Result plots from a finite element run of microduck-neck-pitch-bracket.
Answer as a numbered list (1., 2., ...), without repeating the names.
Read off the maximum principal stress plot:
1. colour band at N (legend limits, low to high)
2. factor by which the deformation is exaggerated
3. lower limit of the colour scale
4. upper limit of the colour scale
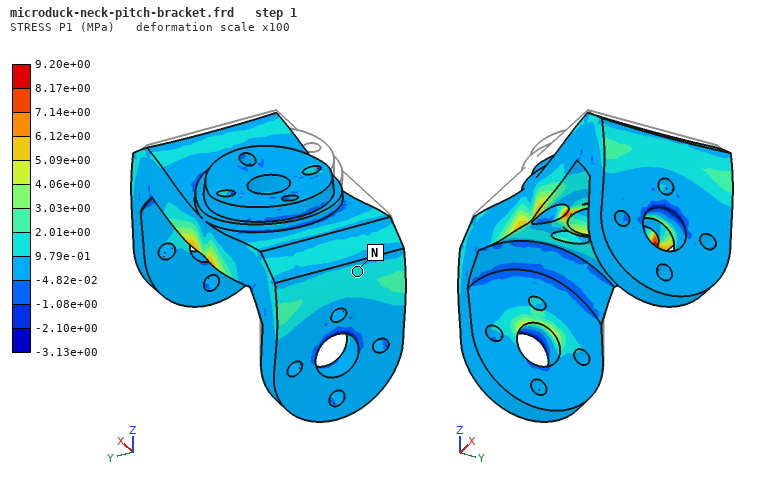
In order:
1. 9.79e-01 to 2.01e+00 MPa
2. 100
3. -3.13e+00 MPa
4. 9.20e+00 MPa
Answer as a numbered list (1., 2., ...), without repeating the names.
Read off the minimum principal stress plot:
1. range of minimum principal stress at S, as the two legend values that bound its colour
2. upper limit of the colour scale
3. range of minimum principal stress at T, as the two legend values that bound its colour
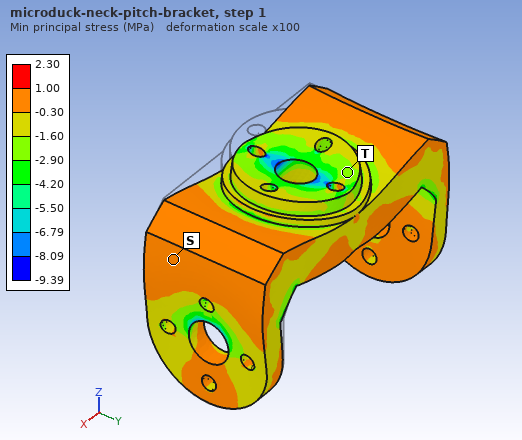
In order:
1. -0.30 to 1.00 MPa
2. 2.30 MPa
3. -2.90 to -1.60 MPa
